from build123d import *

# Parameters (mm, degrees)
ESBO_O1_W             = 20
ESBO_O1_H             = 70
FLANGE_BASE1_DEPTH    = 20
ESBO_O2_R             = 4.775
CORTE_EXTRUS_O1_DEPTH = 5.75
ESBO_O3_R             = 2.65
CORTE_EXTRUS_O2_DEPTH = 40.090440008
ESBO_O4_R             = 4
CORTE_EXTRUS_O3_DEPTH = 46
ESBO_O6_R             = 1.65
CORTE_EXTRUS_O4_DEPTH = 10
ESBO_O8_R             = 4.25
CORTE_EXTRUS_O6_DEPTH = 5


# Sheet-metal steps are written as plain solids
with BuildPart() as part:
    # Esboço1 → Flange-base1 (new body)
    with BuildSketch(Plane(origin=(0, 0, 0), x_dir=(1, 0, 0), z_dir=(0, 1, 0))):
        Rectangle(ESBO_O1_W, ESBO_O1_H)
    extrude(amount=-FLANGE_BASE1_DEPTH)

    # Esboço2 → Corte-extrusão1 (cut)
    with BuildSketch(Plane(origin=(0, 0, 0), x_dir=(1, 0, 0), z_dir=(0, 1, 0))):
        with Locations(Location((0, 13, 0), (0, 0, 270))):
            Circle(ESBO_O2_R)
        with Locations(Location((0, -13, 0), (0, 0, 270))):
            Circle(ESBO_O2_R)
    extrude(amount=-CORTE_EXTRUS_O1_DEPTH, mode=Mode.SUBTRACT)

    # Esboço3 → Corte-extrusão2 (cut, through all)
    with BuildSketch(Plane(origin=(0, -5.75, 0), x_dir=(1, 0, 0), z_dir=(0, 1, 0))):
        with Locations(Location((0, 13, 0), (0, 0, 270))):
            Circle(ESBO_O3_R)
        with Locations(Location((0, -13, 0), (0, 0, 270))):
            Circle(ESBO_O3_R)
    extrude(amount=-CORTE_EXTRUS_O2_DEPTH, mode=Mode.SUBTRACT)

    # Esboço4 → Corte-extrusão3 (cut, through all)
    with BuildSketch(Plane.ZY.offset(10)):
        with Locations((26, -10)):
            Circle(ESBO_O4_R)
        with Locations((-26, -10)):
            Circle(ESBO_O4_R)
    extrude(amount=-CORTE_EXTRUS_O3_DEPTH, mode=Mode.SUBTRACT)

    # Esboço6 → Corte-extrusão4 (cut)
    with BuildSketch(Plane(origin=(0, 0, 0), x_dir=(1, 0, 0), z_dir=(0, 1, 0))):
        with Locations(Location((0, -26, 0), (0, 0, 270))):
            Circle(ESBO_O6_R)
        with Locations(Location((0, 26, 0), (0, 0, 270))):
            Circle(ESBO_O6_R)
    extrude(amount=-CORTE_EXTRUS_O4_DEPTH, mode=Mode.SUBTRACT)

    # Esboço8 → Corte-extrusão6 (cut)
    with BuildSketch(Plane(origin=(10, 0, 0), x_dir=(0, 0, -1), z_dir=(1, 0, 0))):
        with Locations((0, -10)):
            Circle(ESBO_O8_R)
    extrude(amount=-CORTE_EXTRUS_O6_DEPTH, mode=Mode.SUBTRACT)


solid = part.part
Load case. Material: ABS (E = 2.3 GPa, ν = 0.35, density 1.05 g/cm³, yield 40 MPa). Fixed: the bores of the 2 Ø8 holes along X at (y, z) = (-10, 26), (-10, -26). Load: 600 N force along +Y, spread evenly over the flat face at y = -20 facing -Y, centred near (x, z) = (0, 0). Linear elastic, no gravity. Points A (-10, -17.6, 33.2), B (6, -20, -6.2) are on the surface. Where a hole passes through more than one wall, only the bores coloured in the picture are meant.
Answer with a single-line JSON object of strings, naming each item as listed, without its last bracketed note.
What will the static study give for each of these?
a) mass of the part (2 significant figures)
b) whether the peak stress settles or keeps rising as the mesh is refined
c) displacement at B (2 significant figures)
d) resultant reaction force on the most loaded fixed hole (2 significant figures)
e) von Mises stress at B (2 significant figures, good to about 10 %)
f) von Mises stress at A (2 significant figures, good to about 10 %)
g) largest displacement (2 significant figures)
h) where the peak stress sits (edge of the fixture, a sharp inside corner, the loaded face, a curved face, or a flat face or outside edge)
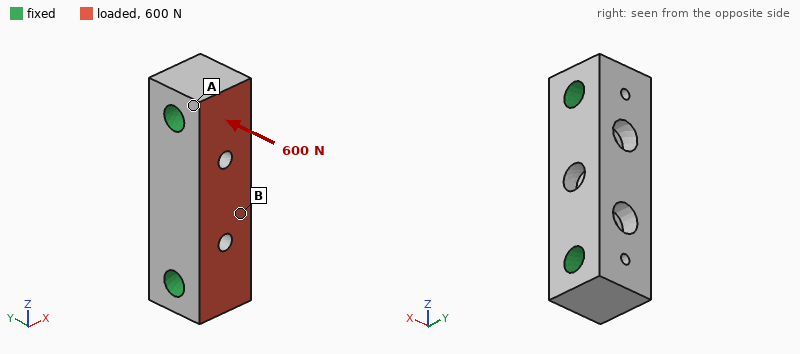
{"mass of the part": "25 g", "whether the peak stress settles or keeps rising as the mesh is refined": "keeps rising", "displacement at B": "16 µm", "resultant reaction force on the most loaded fixed hole": "300 N", "von Mises stress at B": "0.96 MPa", "von Mises stress at A": "0.42 MPa", "largest displacement": "19 µm", "where the peak stress sits": "edge of the fixture"}
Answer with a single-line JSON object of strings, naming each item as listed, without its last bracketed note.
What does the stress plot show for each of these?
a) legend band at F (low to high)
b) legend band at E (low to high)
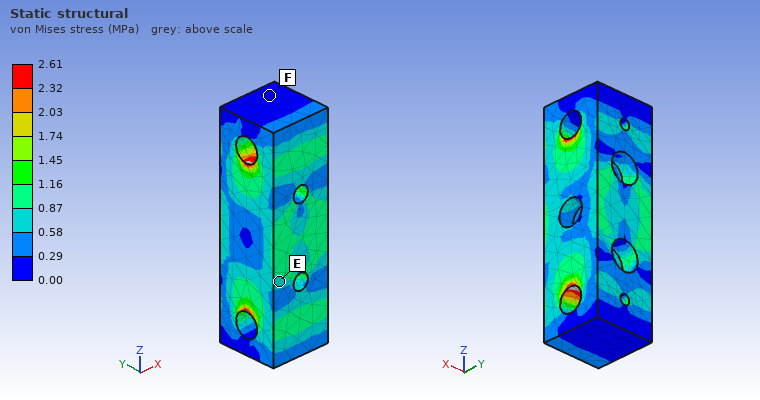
{"legend band at F": "0.00 to 0.29 MPa", "legend band at E": "0.58 to 0.87 MPa"}
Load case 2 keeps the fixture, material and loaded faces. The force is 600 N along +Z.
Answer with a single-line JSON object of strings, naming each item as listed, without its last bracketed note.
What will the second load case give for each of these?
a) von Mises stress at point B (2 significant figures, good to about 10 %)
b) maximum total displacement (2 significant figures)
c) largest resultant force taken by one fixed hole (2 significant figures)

{"von Mises stress at point B": "0.78 MPa", "maximum total displacement": "9.8 µm", "largest resultant force taken by one fixed hole": "310 N"}
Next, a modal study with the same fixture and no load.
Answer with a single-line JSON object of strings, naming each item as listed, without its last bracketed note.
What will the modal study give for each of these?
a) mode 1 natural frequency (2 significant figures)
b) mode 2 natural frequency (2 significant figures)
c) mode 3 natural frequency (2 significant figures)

{"mode 1 natural frequency": "6300 Hz", "mode 2 natural frequency": "6300 Hz", "mode 3 natural frequency": "7900 Hz"}
